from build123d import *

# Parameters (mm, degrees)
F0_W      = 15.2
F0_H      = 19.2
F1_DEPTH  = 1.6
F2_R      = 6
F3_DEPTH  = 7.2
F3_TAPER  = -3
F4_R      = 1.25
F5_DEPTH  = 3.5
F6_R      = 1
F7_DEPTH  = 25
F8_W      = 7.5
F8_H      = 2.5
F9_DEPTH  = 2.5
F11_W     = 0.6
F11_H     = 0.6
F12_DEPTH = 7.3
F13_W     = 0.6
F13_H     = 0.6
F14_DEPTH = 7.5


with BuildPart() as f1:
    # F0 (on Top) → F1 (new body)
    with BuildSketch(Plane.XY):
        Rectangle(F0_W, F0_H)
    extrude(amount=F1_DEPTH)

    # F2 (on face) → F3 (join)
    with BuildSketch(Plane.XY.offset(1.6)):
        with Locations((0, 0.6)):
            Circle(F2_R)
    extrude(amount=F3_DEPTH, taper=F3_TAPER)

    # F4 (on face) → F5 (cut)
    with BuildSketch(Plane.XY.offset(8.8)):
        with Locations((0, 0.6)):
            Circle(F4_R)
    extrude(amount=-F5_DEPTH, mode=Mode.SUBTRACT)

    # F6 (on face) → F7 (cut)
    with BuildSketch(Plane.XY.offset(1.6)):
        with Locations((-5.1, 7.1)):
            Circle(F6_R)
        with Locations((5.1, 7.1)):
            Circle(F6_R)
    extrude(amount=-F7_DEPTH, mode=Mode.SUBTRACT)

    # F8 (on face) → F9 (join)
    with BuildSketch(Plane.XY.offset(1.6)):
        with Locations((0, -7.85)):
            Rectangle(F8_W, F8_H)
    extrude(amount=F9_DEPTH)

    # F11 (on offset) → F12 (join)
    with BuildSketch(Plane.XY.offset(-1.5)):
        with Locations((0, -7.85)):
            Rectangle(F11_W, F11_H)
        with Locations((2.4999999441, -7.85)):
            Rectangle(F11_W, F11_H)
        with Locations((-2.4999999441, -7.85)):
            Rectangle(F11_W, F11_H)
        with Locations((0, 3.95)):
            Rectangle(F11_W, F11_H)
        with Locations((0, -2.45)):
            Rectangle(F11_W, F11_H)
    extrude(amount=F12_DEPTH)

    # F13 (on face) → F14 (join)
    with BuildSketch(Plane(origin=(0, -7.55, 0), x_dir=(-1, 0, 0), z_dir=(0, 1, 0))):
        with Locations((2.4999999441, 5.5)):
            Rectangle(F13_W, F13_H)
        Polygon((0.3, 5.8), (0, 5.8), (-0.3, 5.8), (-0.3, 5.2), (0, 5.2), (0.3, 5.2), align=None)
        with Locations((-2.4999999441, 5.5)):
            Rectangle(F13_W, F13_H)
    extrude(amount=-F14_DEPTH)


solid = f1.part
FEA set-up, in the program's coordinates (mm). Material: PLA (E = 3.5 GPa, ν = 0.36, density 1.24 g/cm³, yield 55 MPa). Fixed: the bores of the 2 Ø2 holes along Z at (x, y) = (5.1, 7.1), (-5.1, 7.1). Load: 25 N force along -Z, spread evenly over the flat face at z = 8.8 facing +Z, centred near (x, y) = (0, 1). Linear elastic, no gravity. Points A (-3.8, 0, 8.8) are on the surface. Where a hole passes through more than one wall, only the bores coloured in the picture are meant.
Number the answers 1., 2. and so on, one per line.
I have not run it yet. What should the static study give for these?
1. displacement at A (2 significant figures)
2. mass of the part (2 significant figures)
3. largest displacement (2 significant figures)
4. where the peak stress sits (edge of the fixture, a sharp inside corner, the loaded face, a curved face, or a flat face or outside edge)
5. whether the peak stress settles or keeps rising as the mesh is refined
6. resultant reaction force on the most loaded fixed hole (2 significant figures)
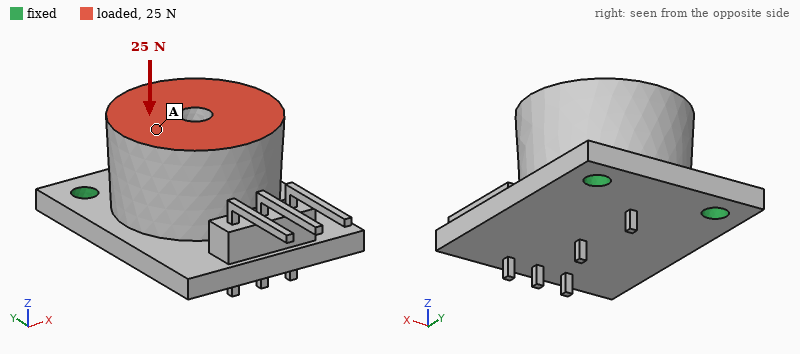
1. 0.15 mm
2. 1.7 g
3. 0.32 mm
4. edge of the fixture
5. keeps rising
6. 13 N
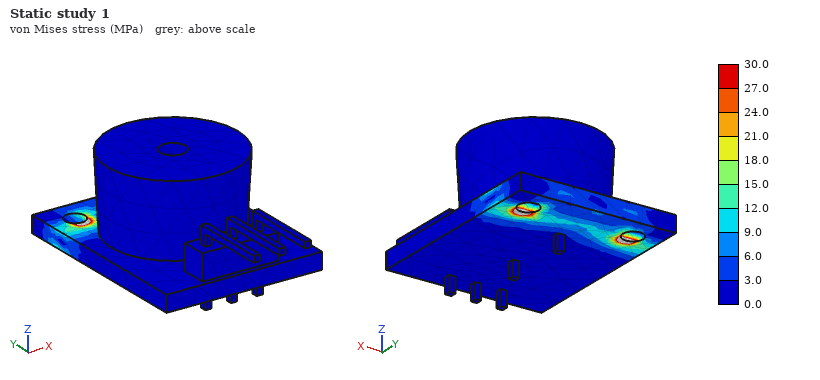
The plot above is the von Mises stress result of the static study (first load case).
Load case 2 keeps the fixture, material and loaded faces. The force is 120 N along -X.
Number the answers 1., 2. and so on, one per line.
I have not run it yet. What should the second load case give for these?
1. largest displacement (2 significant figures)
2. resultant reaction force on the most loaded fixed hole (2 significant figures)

1. 0.15 mm
2. 140 N
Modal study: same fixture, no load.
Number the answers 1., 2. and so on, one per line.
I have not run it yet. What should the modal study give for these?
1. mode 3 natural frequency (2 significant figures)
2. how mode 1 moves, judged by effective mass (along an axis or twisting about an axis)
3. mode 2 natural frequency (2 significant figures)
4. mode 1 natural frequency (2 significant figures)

1. 2200 Hz
2. along Z
3. 2200 Hz
4. 1400 Hz
